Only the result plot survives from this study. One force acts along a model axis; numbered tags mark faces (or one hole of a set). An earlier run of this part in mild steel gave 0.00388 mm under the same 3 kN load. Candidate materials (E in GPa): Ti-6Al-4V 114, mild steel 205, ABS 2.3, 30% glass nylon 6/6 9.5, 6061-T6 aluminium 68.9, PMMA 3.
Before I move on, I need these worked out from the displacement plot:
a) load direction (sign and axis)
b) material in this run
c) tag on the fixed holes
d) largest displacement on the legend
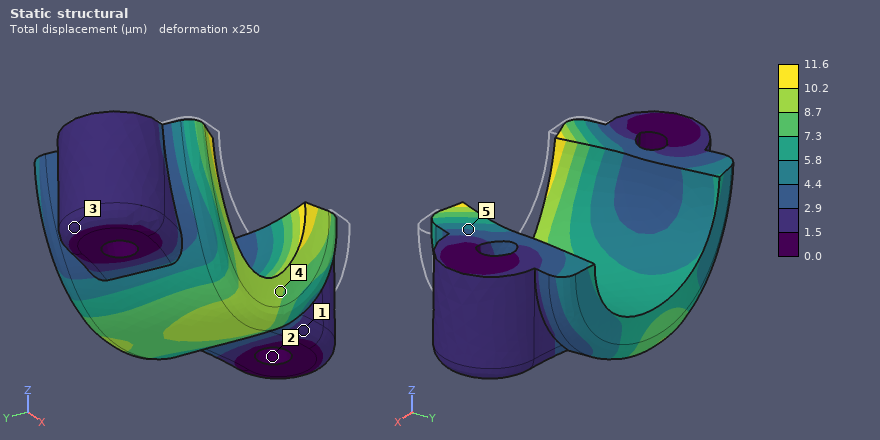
+Y
6061-T6 aluminium
2
11.6 µm
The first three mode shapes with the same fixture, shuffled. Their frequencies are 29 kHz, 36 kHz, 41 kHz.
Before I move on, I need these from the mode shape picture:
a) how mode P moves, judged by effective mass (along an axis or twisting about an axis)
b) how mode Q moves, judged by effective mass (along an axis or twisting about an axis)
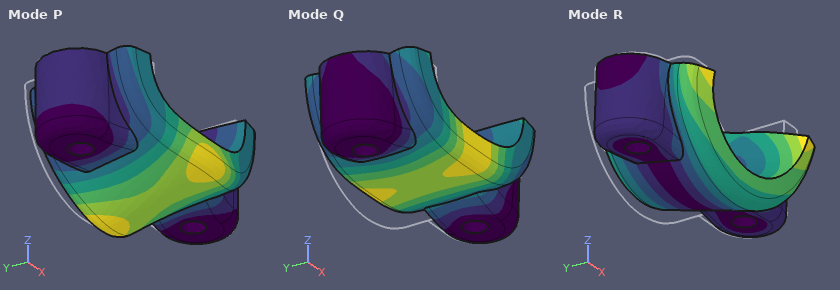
along Y
along Z
